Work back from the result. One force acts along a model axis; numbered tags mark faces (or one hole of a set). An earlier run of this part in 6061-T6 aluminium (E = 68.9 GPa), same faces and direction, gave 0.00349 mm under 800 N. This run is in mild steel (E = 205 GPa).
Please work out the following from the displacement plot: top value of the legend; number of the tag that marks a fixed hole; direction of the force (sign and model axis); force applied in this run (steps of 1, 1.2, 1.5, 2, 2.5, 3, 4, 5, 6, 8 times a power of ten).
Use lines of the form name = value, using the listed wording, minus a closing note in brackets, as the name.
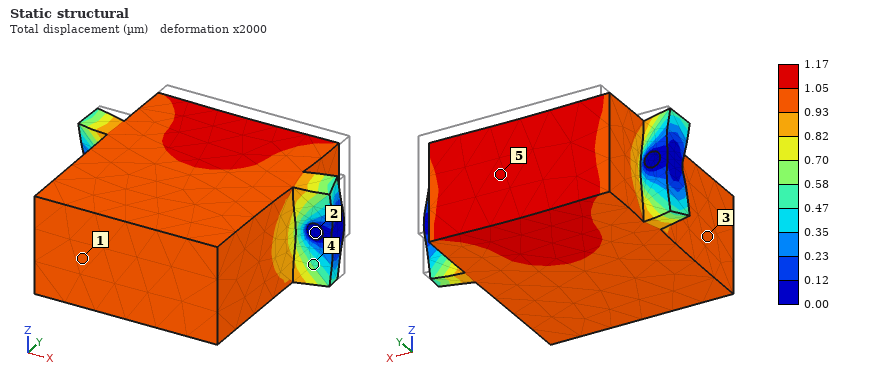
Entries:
top value of the legend = 1.17 µm
number of the tag that marks a fixed hole = 2
direction of the force = -Y
force applied in this run = 800 N
